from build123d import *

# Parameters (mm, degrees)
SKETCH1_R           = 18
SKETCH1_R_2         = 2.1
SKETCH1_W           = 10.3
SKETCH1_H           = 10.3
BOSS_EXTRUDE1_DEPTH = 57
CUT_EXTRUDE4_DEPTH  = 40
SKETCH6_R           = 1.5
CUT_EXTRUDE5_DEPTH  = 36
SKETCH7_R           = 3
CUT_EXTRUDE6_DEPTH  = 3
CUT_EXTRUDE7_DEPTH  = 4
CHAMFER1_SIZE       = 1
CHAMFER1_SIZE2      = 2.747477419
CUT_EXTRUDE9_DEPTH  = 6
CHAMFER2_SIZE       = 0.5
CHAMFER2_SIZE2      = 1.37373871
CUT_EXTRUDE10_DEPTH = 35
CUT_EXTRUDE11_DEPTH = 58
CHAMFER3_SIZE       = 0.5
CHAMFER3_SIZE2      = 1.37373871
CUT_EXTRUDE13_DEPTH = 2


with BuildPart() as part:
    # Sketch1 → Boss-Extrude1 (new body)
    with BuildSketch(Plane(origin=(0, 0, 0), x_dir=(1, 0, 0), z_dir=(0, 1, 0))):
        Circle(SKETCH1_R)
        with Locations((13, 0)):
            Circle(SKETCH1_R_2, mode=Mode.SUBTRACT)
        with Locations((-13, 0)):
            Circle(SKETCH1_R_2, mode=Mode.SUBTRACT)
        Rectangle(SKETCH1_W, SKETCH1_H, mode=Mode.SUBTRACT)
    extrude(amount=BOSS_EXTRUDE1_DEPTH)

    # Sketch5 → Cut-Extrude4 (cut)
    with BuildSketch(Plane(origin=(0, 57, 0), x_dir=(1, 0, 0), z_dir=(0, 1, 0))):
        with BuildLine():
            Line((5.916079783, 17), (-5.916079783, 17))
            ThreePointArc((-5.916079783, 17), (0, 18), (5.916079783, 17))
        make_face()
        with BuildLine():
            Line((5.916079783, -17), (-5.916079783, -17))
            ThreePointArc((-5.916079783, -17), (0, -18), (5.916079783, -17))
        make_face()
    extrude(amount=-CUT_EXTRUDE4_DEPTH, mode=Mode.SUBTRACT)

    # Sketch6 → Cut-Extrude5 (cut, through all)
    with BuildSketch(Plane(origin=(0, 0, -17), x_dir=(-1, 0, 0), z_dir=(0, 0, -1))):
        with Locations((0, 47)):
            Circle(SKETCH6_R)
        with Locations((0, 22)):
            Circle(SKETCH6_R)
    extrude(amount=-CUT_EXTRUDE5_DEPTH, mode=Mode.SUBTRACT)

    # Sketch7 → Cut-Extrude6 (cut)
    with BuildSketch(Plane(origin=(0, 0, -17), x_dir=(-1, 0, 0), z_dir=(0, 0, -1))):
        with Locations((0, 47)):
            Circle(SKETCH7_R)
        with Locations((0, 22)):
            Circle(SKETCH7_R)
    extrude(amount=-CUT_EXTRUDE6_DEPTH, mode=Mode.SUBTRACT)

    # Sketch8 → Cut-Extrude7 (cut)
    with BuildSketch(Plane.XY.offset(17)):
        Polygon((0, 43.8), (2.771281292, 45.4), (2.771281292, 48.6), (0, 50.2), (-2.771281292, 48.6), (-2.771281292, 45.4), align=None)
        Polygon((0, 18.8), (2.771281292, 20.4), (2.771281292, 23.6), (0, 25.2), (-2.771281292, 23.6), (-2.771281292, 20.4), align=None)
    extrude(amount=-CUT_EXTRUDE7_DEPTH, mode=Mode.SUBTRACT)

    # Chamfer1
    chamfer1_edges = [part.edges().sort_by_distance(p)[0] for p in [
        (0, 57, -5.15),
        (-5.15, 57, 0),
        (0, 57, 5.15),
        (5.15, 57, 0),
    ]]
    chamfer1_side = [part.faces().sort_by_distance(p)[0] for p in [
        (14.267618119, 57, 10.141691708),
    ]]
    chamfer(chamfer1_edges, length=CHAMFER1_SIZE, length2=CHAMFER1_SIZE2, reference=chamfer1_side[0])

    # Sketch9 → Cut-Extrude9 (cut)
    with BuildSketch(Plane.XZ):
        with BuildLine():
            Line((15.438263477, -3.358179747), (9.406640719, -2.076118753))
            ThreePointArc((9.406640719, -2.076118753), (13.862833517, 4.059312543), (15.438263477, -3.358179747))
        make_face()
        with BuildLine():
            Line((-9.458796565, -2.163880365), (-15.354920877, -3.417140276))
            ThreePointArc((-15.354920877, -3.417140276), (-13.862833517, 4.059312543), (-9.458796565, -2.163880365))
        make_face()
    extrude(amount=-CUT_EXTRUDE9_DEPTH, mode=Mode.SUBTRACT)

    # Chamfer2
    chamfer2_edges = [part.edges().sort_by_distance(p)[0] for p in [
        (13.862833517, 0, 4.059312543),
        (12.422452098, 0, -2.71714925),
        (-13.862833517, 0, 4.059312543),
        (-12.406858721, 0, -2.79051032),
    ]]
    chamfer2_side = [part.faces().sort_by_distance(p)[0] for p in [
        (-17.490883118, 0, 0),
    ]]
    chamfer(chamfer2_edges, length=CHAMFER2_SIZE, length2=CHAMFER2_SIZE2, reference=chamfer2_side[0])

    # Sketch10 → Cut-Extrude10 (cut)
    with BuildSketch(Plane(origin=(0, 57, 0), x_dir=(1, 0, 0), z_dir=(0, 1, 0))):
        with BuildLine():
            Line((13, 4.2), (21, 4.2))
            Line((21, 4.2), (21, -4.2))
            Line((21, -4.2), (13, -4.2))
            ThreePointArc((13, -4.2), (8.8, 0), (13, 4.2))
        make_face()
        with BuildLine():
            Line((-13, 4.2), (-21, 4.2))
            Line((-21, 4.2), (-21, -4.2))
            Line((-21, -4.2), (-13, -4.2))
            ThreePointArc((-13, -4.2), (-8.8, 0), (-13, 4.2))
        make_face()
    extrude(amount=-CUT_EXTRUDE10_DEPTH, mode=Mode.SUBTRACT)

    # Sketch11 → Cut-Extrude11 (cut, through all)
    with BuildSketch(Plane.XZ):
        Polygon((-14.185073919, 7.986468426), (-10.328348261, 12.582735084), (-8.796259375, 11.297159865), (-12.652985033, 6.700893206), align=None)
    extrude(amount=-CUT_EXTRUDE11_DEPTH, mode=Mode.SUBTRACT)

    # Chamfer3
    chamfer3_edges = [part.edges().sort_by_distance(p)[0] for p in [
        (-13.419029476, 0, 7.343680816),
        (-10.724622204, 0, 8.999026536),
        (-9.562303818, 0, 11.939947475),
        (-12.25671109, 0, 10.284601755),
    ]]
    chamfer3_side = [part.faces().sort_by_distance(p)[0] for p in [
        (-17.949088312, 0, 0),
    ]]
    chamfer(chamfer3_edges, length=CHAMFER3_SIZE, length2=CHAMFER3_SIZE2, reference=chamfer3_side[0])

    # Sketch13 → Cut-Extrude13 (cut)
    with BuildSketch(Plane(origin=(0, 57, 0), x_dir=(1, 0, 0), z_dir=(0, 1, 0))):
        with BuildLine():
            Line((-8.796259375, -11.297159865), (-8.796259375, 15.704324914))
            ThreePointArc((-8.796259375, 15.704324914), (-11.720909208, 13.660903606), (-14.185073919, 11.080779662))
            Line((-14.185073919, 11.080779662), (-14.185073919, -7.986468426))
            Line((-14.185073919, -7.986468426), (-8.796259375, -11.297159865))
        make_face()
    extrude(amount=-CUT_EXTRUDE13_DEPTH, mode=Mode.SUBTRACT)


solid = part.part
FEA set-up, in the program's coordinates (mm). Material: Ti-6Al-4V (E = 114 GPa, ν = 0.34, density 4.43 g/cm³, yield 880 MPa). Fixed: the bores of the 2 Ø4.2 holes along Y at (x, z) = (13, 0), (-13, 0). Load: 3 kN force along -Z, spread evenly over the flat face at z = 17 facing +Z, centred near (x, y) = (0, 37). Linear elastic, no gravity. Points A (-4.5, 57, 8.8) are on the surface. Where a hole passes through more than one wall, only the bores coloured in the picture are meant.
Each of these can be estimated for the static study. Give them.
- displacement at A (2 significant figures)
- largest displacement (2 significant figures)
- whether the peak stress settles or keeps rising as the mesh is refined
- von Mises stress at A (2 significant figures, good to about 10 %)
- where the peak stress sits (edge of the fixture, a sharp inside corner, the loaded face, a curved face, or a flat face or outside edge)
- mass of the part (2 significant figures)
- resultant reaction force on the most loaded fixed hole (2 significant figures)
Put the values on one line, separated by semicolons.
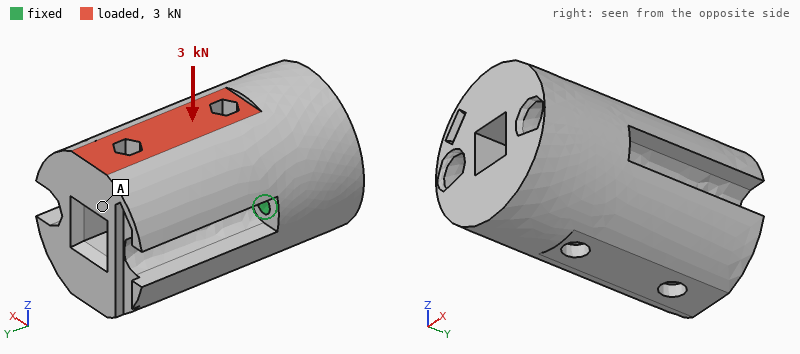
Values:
23 µm; 25 µm; keeps rising; 9.6 MPa; edge of the fixture; 190 g; 1.5 kN
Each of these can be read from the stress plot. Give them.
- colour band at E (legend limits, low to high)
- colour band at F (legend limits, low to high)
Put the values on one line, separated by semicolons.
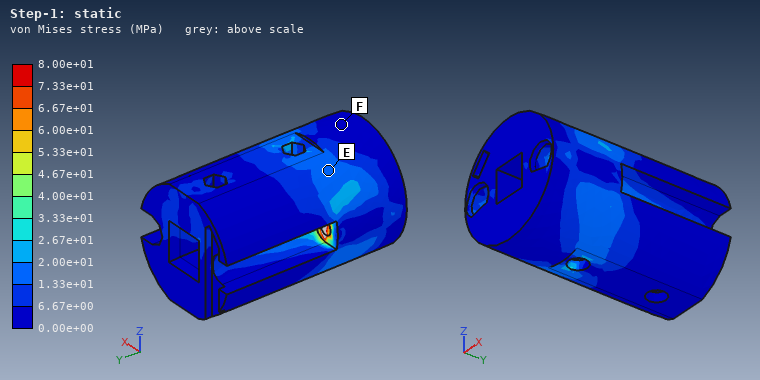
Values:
1.33e+01 to 2.00e+01 MPa; 0.00e+00 to 6.67e+00 MPa
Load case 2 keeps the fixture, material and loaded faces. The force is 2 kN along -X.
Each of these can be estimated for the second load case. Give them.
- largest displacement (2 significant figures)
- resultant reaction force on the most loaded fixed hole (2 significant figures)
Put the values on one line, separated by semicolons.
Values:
10 µm; 2.1 kN
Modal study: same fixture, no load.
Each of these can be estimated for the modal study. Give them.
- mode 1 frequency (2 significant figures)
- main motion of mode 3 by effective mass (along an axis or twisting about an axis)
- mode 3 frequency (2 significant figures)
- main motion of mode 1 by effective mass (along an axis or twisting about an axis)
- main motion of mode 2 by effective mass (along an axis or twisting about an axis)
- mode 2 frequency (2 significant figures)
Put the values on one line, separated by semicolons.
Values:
6000 Hz; twisting about Y; 15 kHz; along Z; along X; 9400 Hz
